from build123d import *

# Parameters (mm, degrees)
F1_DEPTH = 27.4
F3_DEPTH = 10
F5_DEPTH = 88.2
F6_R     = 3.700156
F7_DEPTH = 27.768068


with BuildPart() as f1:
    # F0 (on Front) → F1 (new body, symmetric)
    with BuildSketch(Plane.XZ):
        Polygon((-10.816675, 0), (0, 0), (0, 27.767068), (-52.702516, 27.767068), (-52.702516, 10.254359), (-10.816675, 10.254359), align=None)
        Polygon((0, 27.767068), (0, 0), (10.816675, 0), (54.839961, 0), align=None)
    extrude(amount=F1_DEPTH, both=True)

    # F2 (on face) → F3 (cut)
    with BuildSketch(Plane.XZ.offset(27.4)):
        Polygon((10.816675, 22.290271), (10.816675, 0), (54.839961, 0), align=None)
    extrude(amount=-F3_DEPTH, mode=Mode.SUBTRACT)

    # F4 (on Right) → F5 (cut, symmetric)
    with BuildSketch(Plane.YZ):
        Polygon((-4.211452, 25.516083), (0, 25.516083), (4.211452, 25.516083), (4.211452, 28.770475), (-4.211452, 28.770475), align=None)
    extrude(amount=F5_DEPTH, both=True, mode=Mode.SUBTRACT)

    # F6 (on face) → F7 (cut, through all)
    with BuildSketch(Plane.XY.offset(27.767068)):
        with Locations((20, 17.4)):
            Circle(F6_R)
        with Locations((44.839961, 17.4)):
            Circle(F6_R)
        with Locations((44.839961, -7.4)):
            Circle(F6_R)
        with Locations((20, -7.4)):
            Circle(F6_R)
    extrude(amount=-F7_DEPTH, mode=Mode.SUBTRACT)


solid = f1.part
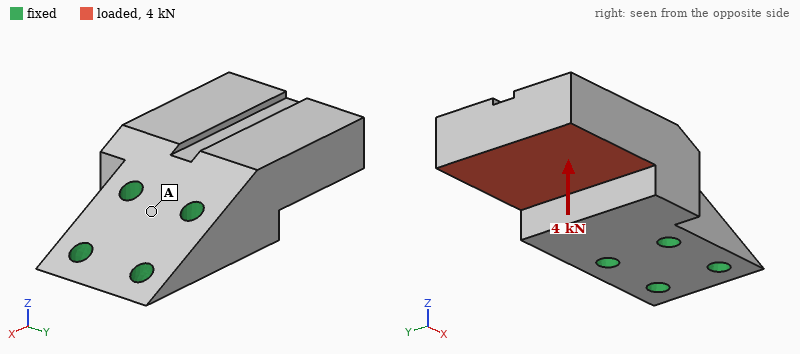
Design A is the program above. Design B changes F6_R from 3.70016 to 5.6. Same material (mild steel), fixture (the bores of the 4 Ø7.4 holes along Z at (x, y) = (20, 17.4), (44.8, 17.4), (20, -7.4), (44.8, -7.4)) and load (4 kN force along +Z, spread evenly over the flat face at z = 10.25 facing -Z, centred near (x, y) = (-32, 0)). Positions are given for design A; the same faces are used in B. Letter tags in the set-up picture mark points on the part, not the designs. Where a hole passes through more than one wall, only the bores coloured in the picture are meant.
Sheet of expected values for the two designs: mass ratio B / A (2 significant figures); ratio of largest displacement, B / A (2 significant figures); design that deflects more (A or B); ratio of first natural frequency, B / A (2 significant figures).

0.97
0.81
A
1.1
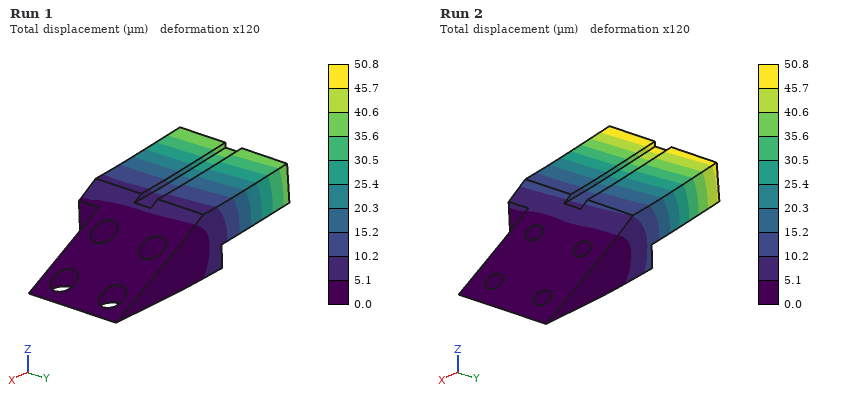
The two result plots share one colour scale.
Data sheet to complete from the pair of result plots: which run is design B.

Run 1
